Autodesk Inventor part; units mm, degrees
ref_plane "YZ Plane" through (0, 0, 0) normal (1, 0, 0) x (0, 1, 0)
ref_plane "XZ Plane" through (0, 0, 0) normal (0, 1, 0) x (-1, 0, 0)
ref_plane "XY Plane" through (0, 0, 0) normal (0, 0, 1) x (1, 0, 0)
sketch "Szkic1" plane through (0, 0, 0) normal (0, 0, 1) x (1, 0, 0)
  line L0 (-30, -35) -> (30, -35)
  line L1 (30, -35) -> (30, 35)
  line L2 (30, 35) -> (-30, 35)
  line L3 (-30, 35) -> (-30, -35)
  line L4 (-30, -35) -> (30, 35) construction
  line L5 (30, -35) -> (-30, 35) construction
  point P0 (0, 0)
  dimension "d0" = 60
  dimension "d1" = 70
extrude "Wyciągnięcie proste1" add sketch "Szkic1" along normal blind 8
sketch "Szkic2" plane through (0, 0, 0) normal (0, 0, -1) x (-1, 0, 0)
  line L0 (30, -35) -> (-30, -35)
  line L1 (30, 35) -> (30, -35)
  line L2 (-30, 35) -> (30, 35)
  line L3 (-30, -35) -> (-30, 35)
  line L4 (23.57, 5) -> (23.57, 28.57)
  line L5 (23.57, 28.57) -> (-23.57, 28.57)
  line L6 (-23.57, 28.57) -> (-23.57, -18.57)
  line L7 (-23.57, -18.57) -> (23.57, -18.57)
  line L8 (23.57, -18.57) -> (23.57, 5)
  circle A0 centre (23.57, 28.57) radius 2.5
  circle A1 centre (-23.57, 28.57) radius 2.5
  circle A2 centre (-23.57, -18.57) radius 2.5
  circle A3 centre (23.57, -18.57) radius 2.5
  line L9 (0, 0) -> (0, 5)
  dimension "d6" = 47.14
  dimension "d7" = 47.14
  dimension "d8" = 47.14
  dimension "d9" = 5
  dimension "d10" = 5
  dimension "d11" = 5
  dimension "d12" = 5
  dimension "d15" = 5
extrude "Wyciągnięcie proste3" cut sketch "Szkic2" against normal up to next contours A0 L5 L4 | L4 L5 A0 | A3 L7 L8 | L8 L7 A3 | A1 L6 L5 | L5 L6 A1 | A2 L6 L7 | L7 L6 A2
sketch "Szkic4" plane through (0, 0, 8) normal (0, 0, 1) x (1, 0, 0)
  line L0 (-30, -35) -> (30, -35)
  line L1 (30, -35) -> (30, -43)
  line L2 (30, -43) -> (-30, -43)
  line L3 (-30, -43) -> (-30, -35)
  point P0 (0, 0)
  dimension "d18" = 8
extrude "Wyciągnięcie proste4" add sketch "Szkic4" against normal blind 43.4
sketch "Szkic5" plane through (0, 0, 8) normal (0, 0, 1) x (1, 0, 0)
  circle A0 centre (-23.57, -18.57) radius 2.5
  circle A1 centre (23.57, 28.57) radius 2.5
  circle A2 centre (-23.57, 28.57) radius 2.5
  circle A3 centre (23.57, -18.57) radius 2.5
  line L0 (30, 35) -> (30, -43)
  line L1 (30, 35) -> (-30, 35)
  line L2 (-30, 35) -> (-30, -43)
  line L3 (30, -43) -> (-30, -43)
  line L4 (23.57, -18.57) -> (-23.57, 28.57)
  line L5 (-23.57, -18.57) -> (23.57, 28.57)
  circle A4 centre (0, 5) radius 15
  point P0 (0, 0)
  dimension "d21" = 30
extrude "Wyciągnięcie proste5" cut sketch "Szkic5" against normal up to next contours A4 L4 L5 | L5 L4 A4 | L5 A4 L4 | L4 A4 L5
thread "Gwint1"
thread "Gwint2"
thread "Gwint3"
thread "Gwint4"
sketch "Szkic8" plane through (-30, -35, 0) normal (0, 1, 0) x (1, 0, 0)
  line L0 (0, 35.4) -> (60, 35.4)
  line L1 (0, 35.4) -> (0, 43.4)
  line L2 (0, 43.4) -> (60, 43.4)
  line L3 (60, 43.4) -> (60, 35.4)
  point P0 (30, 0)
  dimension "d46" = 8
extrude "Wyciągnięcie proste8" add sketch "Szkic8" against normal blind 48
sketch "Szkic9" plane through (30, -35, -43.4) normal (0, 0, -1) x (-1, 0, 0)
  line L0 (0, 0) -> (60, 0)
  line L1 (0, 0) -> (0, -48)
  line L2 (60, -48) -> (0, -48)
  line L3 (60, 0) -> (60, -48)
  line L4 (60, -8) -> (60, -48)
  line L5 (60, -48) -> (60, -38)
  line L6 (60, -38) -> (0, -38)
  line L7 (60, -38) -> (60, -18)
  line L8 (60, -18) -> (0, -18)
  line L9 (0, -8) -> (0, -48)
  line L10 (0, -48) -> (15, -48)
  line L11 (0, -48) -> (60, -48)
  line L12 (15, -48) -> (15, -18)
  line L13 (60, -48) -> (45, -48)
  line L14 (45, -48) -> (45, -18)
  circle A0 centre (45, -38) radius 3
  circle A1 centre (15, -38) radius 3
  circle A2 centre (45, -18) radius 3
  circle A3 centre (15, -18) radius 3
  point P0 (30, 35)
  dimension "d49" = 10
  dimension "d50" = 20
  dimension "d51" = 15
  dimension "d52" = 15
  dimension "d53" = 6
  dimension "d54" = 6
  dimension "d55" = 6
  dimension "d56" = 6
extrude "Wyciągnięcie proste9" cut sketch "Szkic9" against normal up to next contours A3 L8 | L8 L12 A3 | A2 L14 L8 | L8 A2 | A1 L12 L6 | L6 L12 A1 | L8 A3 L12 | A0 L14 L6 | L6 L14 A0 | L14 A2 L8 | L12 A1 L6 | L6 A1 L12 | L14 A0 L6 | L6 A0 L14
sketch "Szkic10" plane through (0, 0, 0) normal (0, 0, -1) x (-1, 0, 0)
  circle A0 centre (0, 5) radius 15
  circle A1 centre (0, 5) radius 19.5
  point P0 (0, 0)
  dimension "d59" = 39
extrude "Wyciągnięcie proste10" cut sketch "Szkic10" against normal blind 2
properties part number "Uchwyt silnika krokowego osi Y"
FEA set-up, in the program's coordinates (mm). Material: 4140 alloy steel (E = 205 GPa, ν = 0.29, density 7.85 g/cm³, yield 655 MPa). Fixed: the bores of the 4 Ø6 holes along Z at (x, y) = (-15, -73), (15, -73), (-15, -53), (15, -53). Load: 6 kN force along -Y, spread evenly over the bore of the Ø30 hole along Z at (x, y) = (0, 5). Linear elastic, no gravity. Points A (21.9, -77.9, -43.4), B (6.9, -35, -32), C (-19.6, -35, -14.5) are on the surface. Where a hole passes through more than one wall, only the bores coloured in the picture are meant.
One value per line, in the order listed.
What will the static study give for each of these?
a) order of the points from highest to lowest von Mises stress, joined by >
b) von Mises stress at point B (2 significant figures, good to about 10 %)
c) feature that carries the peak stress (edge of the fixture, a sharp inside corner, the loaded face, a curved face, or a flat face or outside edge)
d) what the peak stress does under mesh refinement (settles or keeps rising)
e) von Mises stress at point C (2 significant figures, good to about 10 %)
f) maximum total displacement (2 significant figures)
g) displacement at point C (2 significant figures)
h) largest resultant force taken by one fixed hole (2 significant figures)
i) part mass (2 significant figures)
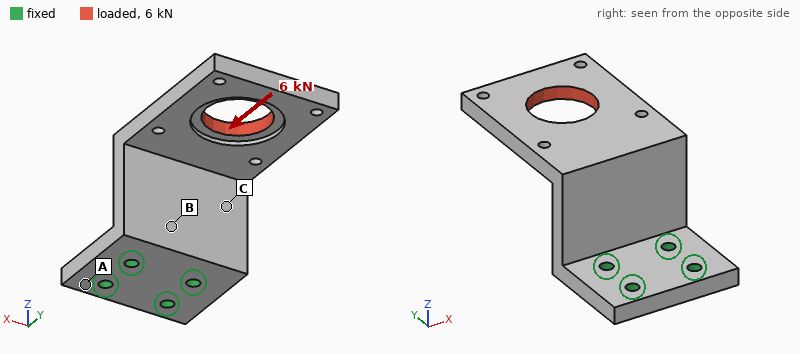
B > C > A
310 MPa
edge of the fixture
keeps rising
180 MPa
1.4 mm
0.29 mm
3.4 kN
540 g
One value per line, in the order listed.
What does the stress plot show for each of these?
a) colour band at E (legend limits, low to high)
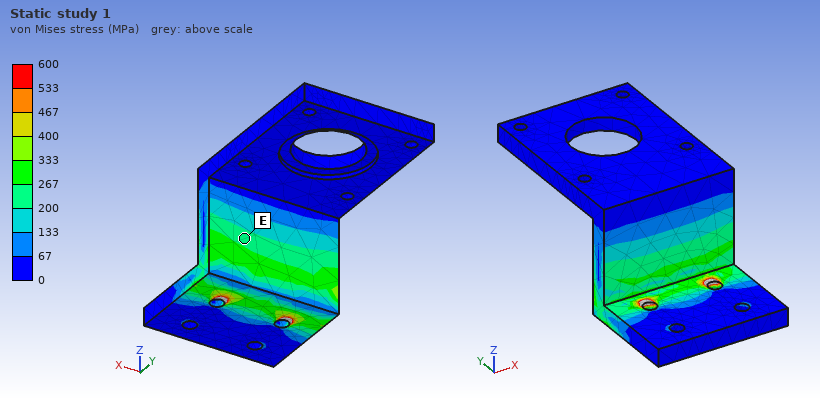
200 to 267 MPa
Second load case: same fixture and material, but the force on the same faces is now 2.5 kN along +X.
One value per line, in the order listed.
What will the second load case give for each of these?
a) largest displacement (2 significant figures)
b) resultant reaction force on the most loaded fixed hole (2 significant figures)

0.31 mm
4.5 kN
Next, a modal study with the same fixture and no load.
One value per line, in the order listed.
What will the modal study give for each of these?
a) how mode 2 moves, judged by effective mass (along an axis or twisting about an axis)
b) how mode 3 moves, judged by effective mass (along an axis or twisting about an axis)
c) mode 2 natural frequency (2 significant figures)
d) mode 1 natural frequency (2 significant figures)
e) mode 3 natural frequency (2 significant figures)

along X
along Y
1200 Hz
580 Hz
1700 Hz
